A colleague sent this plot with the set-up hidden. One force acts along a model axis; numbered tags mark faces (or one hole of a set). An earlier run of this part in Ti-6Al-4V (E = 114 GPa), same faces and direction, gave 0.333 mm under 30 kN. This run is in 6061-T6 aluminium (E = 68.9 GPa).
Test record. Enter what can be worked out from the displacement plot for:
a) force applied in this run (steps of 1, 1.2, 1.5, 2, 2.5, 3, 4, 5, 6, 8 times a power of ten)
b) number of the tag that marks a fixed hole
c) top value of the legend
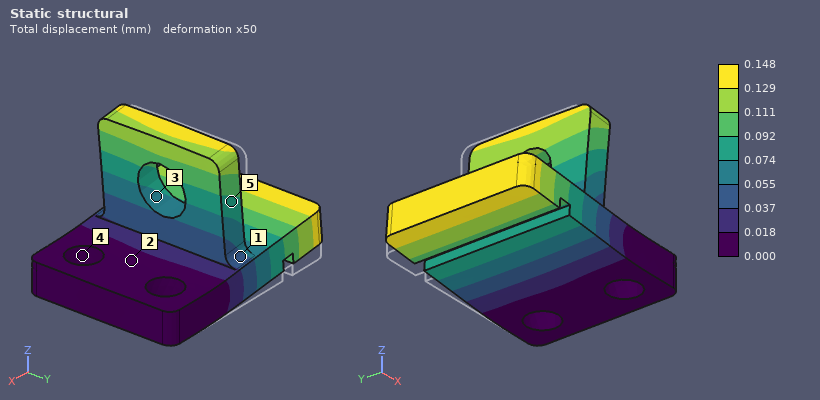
8 kN
4
0.148 mm
